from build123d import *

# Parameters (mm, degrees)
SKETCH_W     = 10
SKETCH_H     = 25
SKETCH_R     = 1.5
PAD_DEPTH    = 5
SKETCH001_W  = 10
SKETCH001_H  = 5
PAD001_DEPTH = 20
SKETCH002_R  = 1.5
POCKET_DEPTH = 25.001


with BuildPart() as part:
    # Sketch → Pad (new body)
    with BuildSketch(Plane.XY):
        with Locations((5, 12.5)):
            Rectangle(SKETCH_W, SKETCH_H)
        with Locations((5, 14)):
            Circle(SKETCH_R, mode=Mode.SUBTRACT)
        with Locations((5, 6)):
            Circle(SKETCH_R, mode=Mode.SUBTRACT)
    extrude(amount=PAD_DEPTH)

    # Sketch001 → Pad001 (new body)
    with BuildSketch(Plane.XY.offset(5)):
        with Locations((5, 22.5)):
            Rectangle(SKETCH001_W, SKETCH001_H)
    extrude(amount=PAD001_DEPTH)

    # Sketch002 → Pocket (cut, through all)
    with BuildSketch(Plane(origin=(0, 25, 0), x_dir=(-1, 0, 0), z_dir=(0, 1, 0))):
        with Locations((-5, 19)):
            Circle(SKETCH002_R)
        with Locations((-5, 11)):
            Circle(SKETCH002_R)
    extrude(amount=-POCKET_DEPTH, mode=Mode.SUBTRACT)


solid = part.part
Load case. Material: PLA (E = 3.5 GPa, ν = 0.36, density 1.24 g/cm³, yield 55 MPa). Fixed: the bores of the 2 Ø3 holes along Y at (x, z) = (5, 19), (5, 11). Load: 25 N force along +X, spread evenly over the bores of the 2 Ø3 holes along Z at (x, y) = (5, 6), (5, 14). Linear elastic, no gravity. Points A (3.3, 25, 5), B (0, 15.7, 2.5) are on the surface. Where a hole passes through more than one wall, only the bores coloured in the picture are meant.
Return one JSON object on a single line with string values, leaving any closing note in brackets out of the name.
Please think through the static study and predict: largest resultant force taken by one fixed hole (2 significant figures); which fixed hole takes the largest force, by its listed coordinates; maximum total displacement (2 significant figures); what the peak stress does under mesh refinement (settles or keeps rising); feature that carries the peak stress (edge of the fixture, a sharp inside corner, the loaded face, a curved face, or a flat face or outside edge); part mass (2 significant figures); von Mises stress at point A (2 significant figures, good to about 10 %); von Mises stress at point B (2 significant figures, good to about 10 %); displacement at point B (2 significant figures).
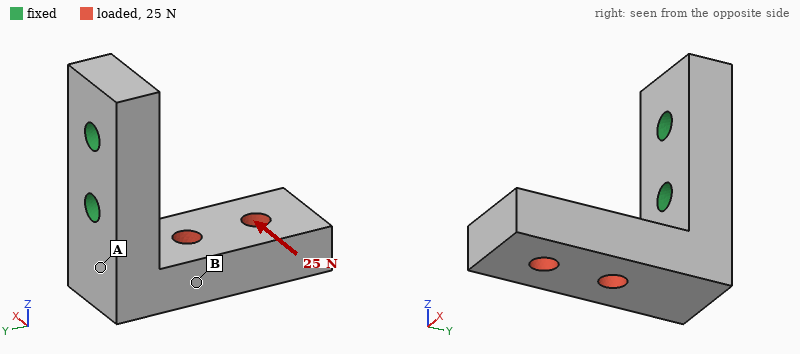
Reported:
{"largest resultant force taken by one fixed hole": "37 N", "which fixed hole takes the largest force, by its listed coordinates": "(5, 11)", "maximum total displacement": "0.16 mm", "what the peak stress does under mesh refinement": "keeps rising", "feature that carries the peak stress": "edge of the fixture", "part mass": "2.6 g", "von Mises stress at point A": "4.0 MPa", "von Mises stress at point B": "2.1 MPa", "displacement at point B": "0.057 mm"}
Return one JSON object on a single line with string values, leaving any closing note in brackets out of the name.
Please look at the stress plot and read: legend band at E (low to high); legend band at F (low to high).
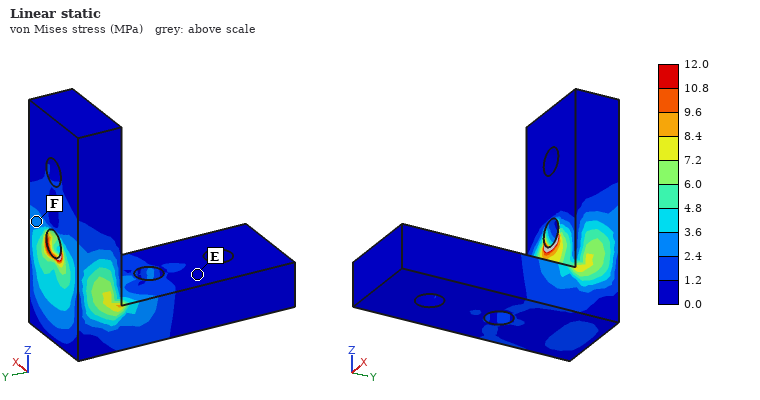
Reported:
{"legend band at E": "0.0 to 1.2 MPa", "legend band at F": "2.4 to 3.6 MPa"}
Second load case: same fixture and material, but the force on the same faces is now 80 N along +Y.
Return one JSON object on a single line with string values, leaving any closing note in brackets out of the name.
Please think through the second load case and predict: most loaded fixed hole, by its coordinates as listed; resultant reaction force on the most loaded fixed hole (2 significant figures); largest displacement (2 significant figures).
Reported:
{"most loaded fixed hole, by its coordinates as listed": "(5, 11)", "resultant reaction force on the most loaded fixed hole": "94 N", "largest displacement": "0.19 mm"}
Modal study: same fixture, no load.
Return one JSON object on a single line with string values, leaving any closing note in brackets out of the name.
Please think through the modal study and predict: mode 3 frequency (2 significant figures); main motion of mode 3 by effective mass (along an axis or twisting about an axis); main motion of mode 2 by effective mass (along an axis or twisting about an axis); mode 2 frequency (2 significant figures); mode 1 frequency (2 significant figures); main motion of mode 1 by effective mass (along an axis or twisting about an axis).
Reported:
{"mode 3 frequency": "6400 Hz", "main motion of mode 3 by effective mass": "along Y", "main motion of mode 2 by effective mass": "along X", "mode 2 frequency": "2200 Hz", "mode 1 frequency": "1800 Hz", "main motion of mode 1 by effective mass": "along Z"}
